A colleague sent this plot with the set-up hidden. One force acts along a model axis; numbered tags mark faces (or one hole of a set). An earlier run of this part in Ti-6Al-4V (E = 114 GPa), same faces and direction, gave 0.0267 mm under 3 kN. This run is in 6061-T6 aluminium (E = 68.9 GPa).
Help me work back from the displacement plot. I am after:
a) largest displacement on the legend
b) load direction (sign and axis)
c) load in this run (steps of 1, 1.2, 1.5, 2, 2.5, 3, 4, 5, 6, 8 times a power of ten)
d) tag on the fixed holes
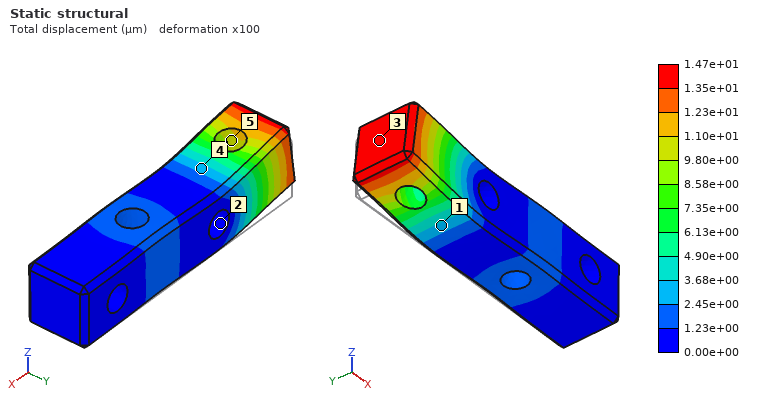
1.47e+01 µm
+Z
1 kN
2
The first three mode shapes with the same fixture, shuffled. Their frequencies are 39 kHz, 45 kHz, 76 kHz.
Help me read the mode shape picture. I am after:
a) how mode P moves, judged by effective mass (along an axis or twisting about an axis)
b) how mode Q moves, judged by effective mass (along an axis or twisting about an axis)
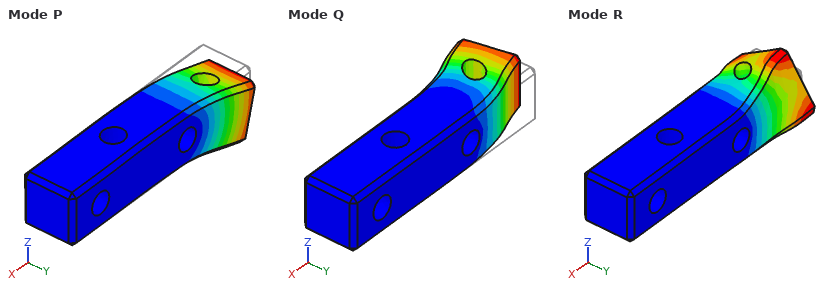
along Z
along Y
